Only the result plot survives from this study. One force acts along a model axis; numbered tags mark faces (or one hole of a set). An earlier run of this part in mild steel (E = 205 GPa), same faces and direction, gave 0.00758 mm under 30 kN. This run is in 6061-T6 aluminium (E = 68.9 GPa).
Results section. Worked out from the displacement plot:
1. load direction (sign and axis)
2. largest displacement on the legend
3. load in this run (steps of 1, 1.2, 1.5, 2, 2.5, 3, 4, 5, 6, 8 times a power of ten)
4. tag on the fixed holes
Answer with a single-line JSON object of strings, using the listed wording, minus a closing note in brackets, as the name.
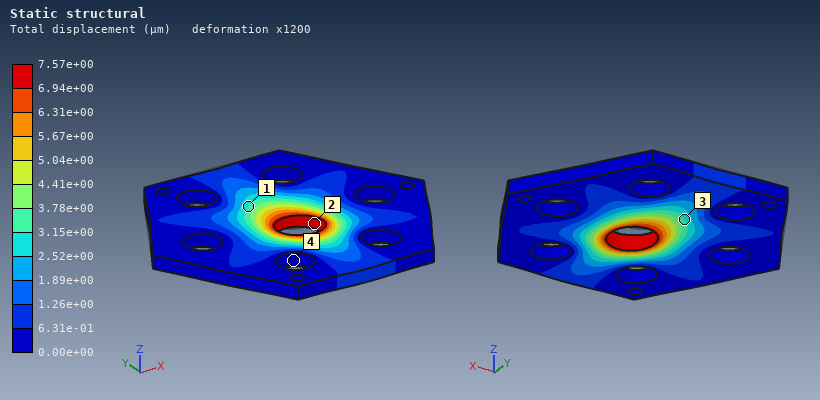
{"load direction": "-Y", "largest displacement on the legend": "7.57e+00 µm", "load in this run": "10 kN", "tag on the fixed holes": "4"}
